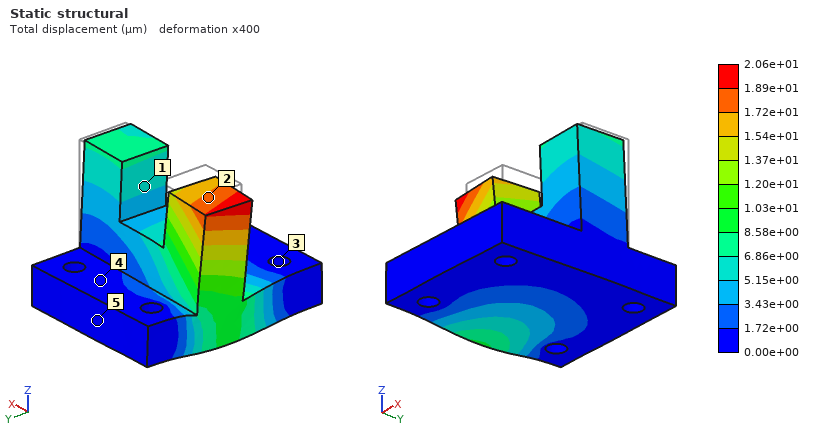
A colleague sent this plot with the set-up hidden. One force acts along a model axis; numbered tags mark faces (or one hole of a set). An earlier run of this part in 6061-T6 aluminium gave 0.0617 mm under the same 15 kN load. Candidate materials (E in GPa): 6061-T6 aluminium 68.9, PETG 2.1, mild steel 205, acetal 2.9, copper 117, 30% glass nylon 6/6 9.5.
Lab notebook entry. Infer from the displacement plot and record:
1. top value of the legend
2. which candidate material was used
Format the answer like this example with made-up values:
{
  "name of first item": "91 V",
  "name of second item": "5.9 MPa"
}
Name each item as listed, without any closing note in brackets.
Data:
{
  "top value of the legend": "2.06e+01 µm",
  "which candidate material was used": "mild steel"
}
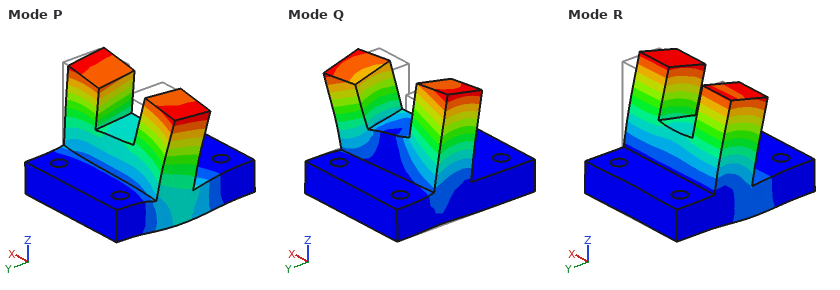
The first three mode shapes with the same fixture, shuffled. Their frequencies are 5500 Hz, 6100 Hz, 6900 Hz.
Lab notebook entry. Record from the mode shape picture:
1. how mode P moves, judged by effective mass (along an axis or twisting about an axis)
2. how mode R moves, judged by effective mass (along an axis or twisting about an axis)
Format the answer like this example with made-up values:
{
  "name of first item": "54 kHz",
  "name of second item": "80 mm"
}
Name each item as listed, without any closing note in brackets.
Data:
{
  "how mode P moves, judged by effective mass": "along X",
  "how mode R moves, judged by effective mass": "along Y"
}
